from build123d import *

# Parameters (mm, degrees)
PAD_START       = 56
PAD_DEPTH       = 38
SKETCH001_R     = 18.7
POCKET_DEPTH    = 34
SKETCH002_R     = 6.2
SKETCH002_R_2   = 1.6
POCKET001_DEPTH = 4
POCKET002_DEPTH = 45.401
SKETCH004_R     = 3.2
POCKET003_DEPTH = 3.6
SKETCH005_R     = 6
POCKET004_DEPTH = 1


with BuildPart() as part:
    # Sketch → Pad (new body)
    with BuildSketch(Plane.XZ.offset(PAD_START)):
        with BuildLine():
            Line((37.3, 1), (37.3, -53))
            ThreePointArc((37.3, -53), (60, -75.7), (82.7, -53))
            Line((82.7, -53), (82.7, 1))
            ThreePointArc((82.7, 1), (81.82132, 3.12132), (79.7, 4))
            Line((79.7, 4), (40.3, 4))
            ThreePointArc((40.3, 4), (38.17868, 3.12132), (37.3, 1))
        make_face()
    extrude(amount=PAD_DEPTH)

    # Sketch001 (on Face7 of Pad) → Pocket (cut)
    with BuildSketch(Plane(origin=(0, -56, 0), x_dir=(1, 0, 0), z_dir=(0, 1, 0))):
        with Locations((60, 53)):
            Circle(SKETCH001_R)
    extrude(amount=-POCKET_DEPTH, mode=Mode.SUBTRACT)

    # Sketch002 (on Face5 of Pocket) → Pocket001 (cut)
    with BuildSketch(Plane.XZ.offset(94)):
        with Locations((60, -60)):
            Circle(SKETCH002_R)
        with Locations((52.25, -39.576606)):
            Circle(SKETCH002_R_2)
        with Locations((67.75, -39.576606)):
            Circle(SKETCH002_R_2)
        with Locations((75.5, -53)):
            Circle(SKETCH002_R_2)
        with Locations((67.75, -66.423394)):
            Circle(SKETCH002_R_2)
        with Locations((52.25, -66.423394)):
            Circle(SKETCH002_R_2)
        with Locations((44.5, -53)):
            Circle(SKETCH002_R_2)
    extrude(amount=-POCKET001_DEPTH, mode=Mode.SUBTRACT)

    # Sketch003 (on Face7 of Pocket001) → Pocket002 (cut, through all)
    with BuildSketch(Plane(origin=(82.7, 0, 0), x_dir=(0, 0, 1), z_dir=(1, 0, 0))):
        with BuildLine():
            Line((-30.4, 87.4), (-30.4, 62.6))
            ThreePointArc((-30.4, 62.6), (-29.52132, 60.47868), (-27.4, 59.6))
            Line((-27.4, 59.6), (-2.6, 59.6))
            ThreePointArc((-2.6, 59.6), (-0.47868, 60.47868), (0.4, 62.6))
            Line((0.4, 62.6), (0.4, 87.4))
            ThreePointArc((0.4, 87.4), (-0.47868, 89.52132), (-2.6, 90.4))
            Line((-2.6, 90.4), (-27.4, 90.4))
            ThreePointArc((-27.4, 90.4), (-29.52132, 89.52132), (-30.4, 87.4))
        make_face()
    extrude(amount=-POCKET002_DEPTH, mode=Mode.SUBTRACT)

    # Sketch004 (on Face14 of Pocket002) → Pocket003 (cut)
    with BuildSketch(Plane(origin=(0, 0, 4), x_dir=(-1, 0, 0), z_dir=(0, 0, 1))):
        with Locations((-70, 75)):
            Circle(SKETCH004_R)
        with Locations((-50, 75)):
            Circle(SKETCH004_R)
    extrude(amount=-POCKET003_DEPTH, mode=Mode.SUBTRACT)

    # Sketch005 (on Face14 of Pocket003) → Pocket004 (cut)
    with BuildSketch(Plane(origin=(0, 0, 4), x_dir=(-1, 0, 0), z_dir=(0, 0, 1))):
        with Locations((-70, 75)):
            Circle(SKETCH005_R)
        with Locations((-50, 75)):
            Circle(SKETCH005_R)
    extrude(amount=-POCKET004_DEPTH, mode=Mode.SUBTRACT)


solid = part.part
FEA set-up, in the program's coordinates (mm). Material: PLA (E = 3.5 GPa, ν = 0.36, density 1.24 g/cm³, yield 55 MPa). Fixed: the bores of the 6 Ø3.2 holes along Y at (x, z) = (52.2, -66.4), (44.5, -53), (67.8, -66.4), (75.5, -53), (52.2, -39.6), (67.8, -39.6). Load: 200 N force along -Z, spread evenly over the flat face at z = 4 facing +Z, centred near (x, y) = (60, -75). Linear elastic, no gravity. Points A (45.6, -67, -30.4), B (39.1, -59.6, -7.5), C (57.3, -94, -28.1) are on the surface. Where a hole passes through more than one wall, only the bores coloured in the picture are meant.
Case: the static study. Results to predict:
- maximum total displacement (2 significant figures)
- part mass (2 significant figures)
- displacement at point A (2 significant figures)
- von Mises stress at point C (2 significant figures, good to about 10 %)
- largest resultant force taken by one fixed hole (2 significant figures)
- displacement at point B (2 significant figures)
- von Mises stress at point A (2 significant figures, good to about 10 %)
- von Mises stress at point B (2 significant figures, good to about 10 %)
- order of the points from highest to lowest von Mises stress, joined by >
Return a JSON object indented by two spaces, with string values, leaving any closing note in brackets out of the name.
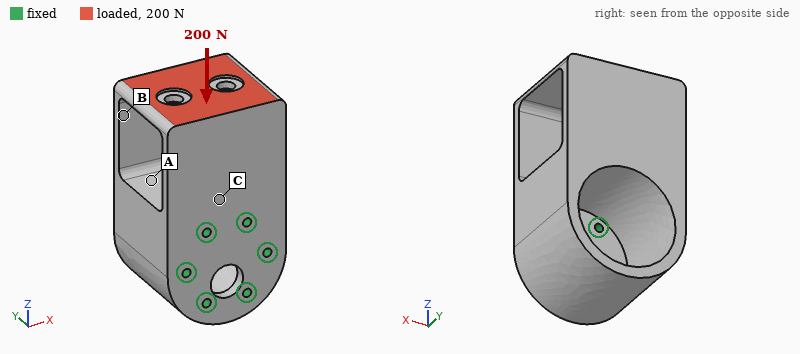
{
  "maximum total displacement": "0.11 mm",
  "part mass": "59 g",
  "displacement at point A": "0.032 mm",
  "von Mises stress at point C": "1.8 MPa",
  "largest resultant force taken by one fixed hole": "75 N",
  "displacement at point B": "0.082 mm",
  "von Mises stress at point A": "0.64 MPa",
  "von Mises stress at point B": "2.8 MPa",
  "order of the points from highest to lowest von Mises stress, joined by >": "B > C > A"
}
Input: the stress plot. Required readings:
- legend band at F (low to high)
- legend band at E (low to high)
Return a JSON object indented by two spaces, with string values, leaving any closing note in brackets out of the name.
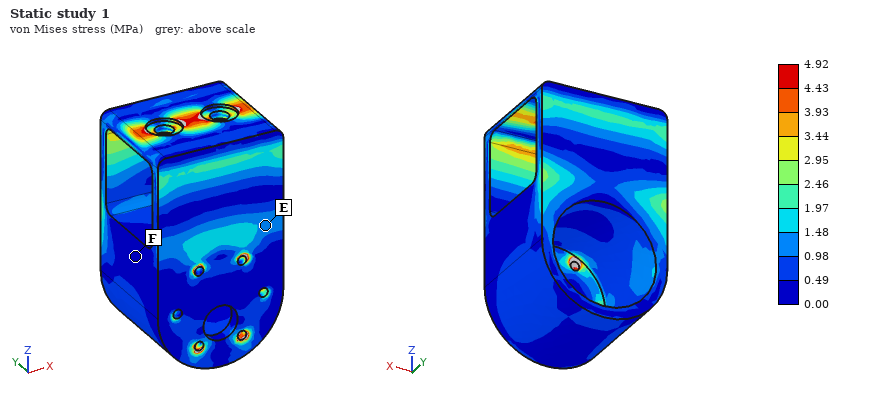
{
  "legend band at F": "0.00 to 0.49 MPa",
  "legend band at E": "0.98 to 1.48 MPa"
}
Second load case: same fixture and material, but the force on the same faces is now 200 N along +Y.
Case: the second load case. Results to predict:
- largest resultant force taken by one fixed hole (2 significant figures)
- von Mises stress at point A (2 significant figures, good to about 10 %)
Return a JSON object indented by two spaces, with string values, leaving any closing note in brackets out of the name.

{
  "largest resultant force taken by one fixed hole": "240 N",
  "von Mises stress at point A": "2.6 MPa"
}
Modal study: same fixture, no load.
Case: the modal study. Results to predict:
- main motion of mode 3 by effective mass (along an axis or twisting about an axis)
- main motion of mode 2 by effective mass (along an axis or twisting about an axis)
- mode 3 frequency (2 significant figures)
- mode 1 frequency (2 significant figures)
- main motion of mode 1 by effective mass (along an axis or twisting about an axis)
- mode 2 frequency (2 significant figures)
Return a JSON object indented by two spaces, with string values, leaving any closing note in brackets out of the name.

{
  "main motion of mode 3 by effective mass": "along Z",
  "main motion of mode 2 by effective mass": "along X",
  "mode 3 frequency": "1900 Hz",
  "mode 1 frequency": "750 Hz",
  "main motion of mode 1 by effective mass": "along Y",
  "mode 2 frequency": "1600 Hz"
}
